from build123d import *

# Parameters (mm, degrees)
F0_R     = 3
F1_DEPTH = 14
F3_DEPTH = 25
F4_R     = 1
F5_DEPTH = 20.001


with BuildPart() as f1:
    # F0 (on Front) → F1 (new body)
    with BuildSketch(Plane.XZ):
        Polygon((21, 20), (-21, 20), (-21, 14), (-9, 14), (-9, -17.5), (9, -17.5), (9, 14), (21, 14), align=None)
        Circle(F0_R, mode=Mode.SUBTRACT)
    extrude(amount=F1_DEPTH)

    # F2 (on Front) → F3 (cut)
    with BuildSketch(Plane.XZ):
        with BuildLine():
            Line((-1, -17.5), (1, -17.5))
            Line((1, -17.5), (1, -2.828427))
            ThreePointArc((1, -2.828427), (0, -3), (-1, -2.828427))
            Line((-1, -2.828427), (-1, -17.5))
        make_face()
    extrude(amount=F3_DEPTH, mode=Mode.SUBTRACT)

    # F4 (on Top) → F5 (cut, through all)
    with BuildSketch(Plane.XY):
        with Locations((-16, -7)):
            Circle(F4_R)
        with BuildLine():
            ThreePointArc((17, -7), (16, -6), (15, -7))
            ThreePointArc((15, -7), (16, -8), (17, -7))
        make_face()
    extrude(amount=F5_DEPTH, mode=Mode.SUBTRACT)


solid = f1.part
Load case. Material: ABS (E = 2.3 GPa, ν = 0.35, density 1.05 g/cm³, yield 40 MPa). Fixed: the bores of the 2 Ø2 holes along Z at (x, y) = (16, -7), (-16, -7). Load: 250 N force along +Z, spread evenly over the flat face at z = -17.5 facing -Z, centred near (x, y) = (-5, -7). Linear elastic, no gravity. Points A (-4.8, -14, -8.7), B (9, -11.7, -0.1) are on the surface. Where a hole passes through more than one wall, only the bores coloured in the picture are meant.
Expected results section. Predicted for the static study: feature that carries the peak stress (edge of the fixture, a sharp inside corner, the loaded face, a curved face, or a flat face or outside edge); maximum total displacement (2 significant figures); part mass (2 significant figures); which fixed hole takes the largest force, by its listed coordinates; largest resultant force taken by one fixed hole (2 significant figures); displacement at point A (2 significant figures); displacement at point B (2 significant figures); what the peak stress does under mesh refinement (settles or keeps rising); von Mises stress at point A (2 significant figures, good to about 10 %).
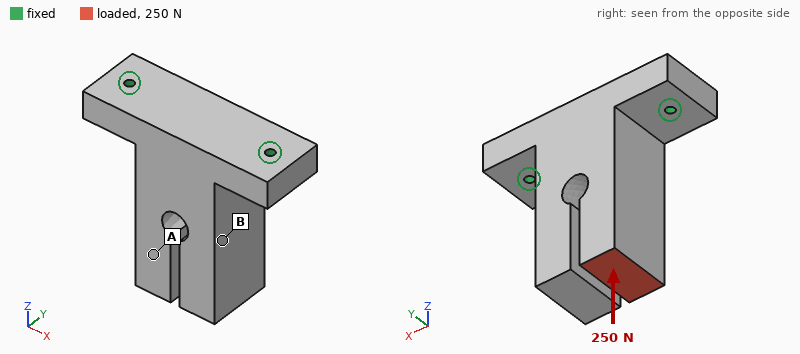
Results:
edge of the fixture
92 µm
11 g
(-16, -7)
180 N
84 µm
42 µm
keeps rising
2.4 MPa
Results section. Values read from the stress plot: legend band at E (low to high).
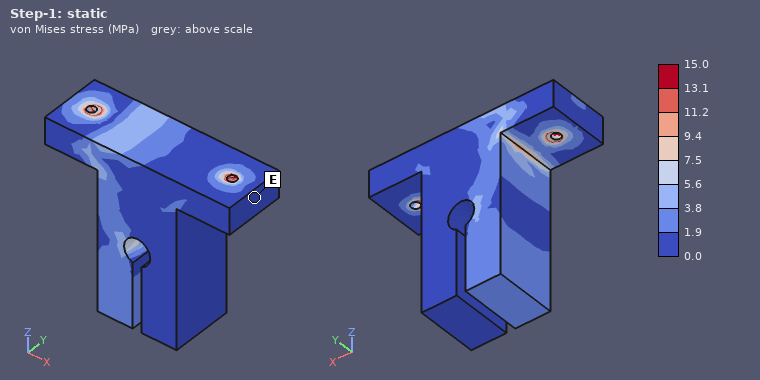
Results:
0.0 to 1.9 MPa
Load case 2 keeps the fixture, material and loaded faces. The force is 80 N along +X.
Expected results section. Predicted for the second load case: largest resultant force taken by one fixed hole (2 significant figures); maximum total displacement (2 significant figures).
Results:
110 N
0.59 mm
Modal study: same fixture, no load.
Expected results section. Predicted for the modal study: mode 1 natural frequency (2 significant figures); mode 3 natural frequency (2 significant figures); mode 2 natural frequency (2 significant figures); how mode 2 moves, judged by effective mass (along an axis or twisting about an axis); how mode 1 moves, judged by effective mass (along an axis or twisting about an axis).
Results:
920 Hz
2400 Hz
1800 Hz
along X
along Y
